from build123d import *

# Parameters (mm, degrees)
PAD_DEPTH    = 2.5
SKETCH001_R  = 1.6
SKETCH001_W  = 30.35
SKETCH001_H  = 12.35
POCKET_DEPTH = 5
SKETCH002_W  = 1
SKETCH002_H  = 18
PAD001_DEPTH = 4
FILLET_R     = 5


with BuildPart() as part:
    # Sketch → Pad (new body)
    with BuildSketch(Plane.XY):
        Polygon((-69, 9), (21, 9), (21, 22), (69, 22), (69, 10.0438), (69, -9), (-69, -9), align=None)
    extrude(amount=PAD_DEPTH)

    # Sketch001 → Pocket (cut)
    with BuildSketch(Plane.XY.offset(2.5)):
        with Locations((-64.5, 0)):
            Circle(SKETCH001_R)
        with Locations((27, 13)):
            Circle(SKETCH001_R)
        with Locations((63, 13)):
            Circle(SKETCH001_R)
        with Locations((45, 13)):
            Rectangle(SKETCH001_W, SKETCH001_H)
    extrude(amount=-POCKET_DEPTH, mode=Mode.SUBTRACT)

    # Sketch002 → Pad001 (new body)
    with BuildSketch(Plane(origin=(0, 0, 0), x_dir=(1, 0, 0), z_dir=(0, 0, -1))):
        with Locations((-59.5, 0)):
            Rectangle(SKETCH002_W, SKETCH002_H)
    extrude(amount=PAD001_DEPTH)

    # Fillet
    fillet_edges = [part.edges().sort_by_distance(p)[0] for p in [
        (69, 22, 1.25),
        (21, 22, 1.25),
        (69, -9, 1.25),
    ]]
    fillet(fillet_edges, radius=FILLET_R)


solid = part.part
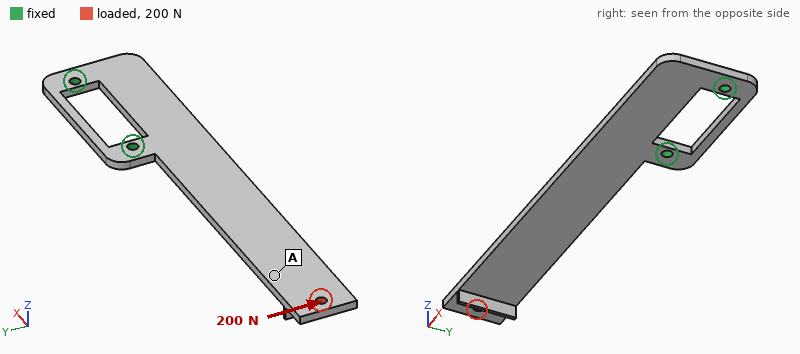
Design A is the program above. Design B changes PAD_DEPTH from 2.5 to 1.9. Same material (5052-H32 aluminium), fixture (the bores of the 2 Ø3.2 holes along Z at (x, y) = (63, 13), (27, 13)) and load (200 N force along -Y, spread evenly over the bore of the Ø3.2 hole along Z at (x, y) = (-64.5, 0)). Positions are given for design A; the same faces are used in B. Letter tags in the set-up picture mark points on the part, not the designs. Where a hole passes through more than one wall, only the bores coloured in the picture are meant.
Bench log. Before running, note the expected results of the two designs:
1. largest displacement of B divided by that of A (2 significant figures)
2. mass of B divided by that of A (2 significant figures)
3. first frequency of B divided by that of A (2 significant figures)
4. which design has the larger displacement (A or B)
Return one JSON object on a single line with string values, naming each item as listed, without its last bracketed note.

{"largest displacement of B divided by that of A": "1.3", "mass of B divided by that of A": "0.76", "first frequency of B divided by that of A": "0.76", "which design has the larger displacement": "B"}
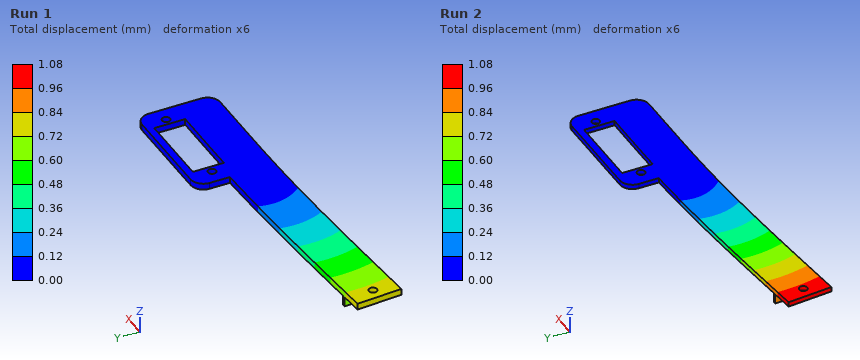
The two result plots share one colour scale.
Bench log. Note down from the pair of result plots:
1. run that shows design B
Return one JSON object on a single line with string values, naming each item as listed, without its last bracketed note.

{"run that shows design B": "Run 2"}
